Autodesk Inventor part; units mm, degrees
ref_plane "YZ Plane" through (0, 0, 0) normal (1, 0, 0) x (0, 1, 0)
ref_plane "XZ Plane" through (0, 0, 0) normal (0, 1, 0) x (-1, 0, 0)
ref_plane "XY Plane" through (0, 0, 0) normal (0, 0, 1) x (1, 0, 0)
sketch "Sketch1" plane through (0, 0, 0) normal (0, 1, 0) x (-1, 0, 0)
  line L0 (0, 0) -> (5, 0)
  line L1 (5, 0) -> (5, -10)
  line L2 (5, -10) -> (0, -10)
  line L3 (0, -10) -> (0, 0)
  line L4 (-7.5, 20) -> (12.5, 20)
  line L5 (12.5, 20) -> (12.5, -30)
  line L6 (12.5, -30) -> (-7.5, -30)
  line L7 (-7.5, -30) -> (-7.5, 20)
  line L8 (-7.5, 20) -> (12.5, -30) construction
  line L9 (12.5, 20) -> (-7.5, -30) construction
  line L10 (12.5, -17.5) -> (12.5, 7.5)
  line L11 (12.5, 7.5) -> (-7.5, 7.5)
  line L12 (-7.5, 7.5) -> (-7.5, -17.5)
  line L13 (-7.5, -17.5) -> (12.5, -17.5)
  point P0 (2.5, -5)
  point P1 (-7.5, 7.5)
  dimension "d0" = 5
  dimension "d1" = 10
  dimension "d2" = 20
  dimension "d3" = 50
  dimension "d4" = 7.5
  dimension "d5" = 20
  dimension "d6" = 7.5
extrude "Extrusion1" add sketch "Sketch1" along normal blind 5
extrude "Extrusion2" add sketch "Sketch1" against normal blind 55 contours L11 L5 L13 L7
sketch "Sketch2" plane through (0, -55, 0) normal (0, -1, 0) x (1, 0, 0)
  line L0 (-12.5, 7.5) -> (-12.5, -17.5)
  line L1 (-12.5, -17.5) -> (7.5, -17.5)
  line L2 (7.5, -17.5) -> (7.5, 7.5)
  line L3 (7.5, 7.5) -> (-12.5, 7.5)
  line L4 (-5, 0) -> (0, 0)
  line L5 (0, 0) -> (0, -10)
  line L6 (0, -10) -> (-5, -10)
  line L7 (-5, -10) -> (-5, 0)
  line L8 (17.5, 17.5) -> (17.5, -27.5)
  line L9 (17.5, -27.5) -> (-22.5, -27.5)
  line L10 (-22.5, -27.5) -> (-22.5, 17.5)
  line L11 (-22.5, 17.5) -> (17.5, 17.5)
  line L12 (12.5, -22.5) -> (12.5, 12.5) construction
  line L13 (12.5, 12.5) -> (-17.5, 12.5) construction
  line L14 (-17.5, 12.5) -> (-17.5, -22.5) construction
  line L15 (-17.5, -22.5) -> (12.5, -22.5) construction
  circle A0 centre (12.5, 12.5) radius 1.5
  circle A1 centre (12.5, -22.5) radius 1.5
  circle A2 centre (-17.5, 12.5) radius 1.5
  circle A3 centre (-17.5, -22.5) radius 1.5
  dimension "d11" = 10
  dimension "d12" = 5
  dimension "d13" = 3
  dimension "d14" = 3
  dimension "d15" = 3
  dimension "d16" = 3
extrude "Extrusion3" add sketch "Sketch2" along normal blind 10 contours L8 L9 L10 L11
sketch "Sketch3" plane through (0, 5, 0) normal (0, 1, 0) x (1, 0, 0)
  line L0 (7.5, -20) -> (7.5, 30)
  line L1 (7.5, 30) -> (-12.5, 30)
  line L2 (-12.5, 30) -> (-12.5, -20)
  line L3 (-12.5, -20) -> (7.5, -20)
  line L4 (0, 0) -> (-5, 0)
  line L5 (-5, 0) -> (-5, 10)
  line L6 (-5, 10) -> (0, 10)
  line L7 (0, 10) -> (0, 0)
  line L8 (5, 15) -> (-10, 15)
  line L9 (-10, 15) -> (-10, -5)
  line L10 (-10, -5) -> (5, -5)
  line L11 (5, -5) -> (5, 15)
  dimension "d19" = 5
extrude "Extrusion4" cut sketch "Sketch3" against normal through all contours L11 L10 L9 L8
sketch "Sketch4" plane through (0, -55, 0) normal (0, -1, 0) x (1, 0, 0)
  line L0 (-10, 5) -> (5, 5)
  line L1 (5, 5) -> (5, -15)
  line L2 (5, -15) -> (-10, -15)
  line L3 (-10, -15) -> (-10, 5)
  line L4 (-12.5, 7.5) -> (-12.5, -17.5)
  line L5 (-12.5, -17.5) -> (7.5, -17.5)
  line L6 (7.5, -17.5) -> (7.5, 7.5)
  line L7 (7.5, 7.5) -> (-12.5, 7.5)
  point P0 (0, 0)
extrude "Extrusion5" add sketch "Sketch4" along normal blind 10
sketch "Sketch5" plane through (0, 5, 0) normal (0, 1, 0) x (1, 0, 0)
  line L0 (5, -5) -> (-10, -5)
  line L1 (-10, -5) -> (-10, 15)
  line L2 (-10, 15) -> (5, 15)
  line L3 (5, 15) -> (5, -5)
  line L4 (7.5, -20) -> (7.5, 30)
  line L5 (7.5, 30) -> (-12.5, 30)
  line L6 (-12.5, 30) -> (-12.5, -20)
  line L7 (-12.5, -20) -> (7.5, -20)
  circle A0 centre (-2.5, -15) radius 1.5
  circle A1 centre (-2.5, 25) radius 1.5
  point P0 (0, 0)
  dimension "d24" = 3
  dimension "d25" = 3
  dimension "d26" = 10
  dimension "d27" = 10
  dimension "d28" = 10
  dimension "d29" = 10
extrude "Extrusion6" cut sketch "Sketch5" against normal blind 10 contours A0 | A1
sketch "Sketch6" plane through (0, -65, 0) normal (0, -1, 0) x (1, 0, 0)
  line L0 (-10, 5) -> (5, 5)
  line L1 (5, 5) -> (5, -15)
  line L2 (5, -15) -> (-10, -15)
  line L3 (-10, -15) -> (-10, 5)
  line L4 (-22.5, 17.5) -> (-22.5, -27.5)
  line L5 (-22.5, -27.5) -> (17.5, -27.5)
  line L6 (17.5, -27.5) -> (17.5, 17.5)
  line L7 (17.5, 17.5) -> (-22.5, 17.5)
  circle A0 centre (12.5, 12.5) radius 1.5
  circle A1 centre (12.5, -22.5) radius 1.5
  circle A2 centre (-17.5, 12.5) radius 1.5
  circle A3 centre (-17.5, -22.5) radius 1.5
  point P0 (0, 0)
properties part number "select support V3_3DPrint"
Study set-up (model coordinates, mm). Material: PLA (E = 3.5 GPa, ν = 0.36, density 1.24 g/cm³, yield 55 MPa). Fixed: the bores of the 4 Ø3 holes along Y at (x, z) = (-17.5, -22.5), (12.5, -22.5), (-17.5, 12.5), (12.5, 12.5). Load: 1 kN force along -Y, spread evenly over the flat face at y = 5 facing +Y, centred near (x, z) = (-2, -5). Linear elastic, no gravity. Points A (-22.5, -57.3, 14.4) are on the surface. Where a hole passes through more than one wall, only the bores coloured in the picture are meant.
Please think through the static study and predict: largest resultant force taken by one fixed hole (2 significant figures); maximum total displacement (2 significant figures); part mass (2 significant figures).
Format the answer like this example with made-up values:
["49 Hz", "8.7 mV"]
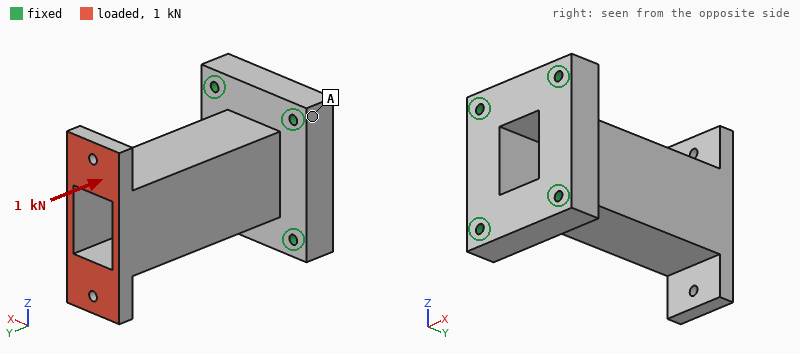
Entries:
["260 N", "0.68 mm", "36 g"]
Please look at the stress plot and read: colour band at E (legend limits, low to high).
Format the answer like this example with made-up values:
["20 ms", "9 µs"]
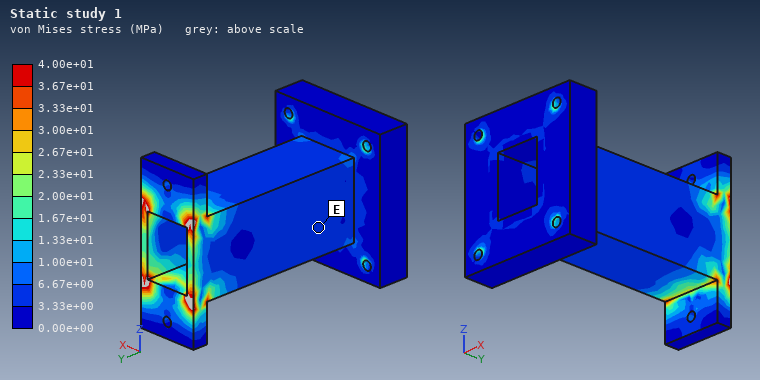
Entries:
["3.33e+00 to 6.67e+00 MPa"]
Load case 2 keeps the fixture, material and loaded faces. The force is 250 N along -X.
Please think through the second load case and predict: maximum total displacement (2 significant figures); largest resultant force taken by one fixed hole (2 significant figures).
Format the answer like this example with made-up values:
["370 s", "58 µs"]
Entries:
["0.93 mm", "320 N"]
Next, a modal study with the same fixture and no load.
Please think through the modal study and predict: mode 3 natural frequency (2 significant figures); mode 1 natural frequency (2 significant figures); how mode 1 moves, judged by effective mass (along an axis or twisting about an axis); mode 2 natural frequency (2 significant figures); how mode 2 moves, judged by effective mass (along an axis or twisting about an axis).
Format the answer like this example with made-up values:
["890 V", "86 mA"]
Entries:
["2300 Hz", "990 Hz", "along X", "1200 Hz", "along Z"]
